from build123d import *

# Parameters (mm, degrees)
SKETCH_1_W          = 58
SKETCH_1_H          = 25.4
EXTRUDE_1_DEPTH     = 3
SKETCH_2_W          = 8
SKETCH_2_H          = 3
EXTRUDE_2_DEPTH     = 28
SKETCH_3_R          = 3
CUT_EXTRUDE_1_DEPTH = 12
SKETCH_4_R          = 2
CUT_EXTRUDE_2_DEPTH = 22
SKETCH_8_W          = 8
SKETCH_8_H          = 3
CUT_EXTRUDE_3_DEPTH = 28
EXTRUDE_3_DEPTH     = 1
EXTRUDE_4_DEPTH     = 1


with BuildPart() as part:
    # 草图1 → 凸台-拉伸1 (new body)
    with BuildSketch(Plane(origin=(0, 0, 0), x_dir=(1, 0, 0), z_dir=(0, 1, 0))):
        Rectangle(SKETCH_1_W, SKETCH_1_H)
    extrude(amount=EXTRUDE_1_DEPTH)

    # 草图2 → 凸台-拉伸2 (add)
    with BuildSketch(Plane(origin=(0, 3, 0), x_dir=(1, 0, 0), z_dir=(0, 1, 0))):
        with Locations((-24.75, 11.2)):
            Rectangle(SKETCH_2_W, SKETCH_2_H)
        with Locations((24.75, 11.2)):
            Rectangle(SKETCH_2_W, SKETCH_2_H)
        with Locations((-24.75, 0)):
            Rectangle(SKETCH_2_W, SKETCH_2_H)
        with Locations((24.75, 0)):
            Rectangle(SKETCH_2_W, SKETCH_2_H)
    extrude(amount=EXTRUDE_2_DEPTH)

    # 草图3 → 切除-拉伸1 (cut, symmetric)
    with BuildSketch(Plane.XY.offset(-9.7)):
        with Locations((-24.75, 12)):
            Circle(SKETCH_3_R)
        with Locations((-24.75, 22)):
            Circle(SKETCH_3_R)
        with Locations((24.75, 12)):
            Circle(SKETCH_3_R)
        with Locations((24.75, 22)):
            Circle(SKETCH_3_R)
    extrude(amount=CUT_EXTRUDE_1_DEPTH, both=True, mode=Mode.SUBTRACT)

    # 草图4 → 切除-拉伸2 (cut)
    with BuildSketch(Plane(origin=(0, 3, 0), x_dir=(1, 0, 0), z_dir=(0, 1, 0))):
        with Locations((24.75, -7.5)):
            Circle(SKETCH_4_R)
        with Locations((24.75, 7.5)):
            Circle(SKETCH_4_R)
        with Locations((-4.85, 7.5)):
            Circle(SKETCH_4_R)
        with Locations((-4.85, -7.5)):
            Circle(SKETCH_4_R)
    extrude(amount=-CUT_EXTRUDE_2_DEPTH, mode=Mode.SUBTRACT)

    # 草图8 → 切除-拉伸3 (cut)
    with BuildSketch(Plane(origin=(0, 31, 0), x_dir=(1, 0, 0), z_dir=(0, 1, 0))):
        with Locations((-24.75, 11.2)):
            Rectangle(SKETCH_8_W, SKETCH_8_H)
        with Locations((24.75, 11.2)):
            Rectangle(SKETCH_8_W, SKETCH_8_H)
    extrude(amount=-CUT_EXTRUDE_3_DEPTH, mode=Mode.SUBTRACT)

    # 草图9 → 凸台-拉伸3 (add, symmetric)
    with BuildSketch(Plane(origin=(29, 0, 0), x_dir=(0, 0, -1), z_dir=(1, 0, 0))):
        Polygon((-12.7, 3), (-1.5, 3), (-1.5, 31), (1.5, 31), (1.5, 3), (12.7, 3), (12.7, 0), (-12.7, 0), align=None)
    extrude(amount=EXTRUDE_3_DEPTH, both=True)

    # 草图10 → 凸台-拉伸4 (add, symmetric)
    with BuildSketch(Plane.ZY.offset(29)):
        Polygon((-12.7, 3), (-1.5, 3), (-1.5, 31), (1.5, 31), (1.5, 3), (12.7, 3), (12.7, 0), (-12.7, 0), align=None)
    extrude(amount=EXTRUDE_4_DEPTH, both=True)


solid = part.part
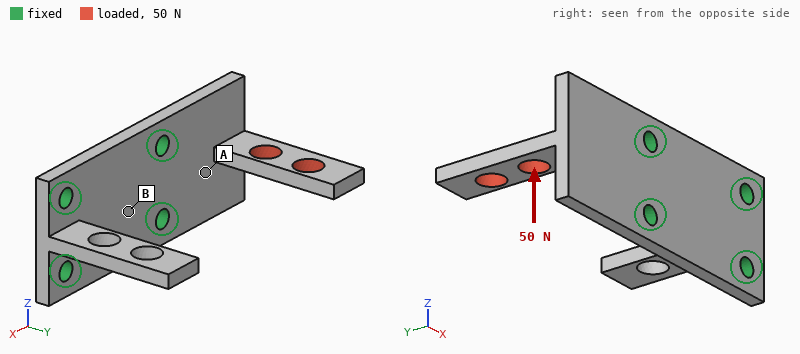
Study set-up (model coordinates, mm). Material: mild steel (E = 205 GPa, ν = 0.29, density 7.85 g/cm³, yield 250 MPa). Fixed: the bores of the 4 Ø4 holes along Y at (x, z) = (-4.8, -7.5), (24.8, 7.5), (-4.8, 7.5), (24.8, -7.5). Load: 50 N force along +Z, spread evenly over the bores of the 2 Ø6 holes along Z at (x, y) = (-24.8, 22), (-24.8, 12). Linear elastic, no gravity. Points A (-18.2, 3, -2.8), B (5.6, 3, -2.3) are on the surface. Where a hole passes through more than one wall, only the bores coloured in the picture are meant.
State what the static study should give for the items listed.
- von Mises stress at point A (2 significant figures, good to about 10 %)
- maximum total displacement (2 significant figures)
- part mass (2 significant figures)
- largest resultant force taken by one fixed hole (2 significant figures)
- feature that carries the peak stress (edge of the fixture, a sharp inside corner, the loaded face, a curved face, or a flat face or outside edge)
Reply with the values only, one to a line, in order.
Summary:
18 MPa
68 µm
44 g
73 N
the loaded face
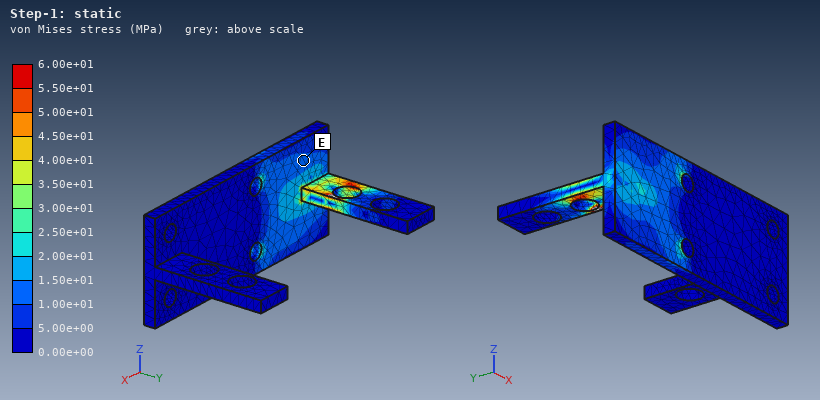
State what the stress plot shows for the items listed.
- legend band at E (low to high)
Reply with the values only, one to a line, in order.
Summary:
1.00e+01 to 1.50e+01 MPa
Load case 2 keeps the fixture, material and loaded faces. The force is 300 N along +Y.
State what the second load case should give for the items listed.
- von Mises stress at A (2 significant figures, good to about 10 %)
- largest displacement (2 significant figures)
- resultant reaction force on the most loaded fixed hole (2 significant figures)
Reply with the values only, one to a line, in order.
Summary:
54 MPa
0.16 mm
160 N
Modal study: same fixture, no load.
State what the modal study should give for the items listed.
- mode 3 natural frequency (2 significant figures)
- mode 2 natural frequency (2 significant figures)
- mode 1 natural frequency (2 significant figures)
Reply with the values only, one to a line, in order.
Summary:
2600 Hz
2300 Hz
2300 Hz
